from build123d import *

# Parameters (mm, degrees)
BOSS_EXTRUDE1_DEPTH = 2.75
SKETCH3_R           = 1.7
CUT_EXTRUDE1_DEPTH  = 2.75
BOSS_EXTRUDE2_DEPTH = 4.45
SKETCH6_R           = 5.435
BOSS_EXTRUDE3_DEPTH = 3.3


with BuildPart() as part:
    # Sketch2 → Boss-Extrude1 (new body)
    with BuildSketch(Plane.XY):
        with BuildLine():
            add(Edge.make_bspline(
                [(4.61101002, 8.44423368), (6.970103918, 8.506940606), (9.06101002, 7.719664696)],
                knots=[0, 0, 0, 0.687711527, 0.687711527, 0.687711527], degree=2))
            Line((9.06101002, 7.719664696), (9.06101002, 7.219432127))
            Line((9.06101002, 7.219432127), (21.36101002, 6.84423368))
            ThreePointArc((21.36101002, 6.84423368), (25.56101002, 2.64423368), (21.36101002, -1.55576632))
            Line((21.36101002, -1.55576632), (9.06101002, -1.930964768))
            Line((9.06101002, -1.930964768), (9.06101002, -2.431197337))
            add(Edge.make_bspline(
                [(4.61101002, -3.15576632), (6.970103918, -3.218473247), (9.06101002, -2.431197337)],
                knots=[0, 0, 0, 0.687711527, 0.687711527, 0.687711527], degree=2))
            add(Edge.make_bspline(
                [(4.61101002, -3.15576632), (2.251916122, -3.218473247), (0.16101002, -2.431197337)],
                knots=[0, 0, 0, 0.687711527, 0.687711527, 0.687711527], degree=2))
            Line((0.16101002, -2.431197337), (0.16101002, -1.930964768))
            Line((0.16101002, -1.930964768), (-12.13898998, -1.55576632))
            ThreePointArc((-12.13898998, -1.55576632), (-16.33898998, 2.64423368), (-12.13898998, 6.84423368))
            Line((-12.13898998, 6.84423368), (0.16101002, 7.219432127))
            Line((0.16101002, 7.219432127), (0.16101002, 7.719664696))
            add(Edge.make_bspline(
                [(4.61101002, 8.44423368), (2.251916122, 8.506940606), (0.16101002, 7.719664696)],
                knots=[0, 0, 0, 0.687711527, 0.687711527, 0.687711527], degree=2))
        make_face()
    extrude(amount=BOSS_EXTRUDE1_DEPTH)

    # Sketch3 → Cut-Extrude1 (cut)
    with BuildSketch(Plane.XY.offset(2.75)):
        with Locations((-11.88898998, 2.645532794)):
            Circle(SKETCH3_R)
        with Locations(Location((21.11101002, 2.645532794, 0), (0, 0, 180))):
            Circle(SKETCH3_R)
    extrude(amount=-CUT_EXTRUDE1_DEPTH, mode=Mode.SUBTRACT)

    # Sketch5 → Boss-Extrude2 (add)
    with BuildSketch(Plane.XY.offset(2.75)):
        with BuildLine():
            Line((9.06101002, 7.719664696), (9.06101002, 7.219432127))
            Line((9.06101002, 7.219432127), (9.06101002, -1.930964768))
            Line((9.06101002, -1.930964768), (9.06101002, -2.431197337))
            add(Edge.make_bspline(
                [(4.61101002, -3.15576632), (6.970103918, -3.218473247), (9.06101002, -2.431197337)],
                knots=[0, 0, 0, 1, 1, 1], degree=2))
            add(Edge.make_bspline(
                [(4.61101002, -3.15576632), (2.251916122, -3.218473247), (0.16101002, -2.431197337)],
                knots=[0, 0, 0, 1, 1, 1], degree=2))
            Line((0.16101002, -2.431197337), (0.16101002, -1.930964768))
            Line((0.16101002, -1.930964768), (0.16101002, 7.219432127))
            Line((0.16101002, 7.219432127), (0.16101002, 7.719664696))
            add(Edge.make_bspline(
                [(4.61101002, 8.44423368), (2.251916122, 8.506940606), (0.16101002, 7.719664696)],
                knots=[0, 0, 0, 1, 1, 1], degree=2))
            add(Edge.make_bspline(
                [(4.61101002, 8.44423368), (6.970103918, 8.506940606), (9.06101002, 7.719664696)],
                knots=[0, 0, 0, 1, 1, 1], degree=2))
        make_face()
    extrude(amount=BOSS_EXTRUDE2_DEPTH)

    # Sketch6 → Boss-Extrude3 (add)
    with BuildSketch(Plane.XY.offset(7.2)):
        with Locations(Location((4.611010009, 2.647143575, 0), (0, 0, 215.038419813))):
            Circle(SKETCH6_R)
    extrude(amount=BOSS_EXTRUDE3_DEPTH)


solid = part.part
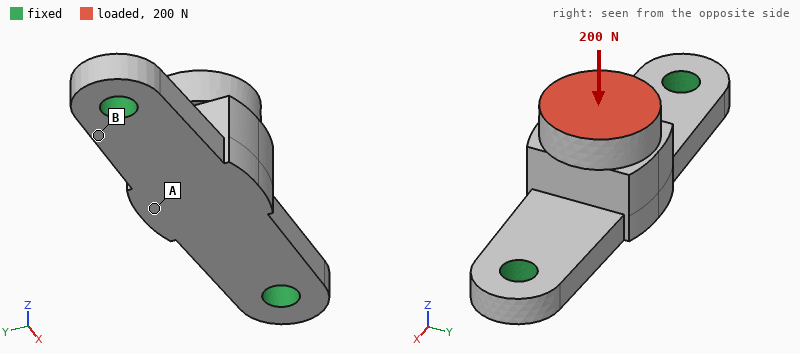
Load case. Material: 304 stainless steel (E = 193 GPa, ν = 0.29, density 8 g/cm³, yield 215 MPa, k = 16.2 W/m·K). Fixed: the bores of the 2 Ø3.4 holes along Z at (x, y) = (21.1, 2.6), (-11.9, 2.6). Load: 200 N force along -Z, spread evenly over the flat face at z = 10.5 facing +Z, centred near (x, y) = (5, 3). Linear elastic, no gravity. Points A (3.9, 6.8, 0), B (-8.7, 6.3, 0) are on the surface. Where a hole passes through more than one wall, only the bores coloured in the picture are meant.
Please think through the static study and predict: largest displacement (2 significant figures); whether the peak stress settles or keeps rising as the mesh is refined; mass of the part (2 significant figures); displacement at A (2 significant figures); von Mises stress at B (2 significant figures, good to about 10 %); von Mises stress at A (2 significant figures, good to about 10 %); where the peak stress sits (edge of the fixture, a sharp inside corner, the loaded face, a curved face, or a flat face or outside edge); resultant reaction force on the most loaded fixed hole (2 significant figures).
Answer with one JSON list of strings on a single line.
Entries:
["6.2 µm", "keeps rising", "14 g", "6.2 µm", "30 MPa", "9.6 MPa", "edge of the fixture", "110 N"]
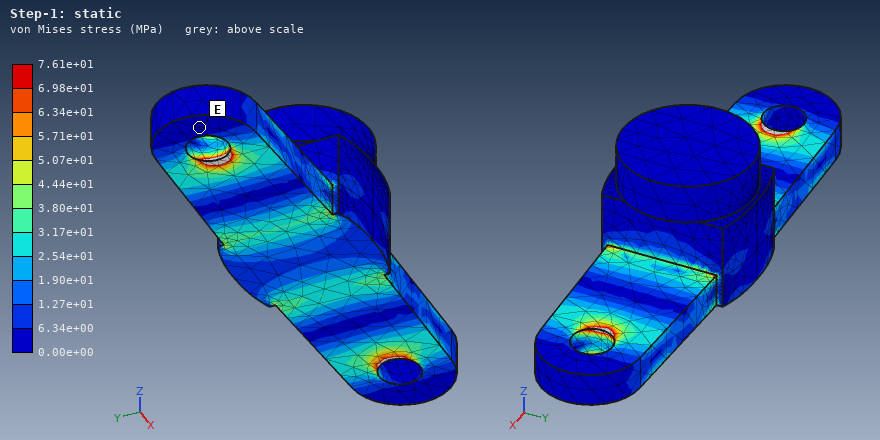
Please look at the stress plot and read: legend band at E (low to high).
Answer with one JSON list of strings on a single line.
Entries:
["0.00e+00 to 6.34e+00 MPa"]
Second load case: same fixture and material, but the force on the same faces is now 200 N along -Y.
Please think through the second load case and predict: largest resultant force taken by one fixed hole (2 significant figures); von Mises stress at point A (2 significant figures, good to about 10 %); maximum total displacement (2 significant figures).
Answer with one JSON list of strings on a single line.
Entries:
["100 N", "23 MPa", "29 µm"]
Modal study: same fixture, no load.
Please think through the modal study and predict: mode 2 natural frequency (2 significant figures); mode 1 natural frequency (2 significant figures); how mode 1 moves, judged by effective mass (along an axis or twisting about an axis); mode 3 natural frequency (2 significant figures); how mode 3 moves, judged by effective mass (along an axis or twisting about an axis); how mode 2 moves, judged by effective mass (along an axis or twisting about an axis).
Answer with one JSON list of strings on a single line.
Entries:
["9300 Hz", "7700 Hz", "along Y", "17 kHz", "along X", "along Z"]
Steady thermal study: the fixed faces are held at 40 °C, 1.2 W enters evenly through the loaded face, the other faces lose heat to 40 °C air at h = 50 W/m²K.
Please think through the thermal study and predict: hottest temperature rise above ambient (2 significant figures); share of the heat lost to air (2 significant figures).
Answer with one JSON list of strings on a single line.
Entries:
["18 K", "40 %"]
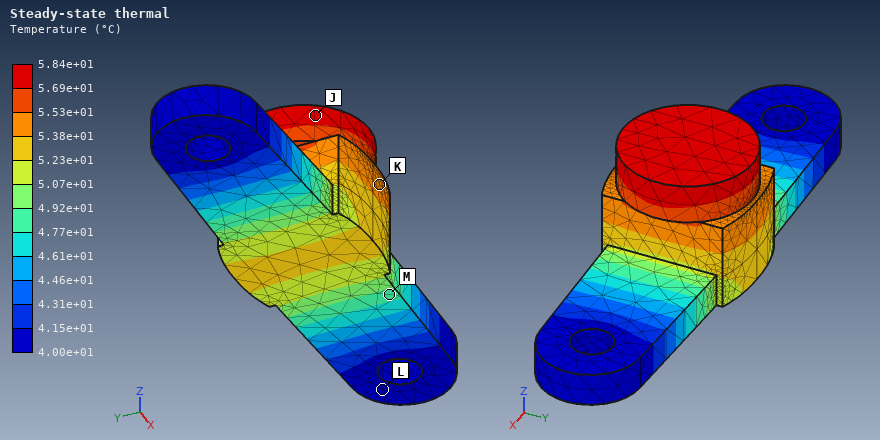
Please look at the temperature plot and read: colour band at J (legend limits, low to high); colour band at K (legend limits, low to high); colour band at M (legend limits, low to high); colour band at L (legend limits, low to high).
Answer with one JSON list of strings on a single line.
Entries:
["5.69e+01 to 5.84e+01 °C", "5.38e+01 to 5.53e+01 °C", "4.77e+01 to 4.92e+01 °C", "4.00e+01 to 4.15e+01 °C"]
